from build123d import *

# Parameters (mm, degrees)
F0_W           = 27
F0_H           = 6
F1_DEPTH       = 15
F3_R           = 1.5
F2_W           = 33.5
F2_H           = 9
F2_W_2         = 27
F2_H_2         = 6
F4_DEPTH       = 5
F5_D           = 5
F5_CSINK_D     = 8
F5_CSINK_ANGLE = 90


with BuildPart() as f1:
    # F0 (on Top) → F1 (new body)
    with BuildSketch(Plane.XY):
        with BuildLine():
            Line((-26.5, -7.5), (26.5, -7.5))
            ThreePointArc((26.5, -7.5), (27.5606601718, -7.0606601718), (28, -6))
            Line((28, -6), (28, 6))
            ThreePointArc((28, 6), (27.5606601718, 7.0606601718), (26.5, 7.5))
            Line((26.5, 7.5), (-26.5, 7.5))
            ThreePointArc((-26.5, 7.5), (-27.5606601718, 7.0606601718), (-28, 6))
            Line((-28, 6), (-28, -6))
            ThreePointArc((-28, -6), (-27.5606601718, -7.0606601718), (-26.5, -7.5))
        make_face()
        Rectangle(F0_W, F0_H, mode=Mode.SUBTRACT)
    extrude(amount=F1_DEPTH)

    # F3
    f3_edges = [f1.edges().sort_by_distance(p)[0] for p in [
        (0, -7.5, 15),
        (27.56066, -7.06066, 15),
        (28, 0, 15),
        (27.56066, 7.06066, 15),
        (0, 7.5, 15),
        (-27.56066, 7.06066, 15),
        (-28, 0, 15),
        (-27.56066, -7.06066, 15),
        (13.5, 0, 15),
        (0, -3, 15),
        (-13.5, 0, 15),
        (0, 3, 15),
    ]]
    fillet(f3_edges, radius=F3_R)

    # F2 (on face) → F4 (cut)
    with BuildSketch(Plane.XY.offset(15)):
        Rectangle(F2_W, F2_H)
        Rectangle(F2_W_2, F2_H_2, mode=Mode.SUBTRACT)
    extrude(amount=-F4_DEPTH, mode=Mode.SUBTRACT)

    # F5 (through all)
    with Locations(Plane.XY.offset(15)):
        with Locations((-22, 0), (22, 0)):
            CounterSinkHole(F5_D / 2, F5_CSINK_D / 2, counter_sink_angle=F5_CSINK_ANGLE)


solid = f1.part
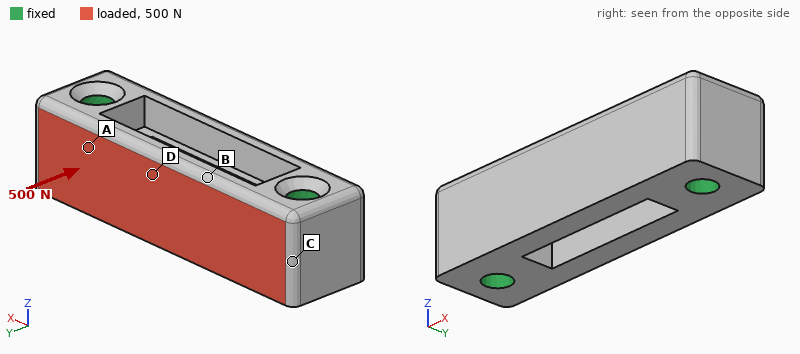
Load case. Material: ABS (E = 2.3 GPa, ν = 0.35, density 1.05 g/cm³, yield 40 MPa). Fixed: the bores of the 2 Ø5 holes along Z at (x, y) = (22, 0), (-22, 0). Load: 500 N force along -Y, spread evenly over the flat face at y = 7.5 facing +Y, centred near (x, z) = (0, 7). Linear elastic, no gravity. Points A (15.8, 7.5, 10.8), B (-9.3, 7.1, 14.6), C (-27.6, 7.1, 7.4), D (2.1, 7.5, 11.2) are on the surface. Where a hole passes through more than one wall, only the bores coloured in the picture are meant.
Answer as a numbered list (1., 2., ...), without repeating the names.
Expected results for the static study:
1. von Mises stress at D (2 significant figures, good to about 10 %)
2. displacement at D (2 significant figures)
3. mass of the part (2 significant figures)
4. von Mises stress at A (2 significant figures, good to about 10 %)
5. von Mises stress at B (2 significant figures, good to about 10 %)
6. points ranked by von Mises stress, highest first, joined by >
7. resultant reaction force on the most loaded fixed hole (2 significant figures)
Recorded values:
1. 9.7 MPa
2. 0.19 mm
3. 9.2 g
4. 7.4 MPa
5. 3.0 MPa
6. D > A > B > C
7. 260 N
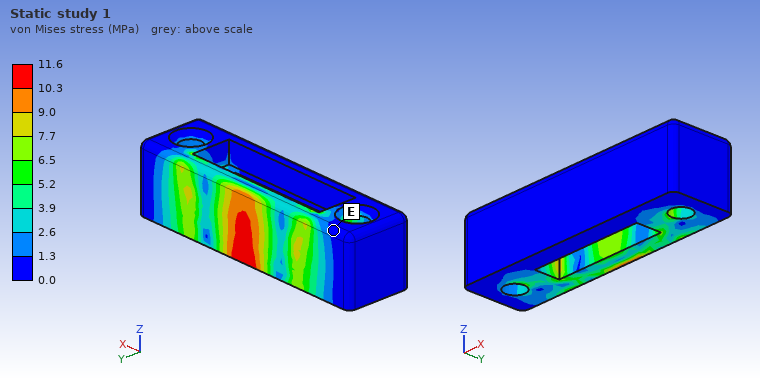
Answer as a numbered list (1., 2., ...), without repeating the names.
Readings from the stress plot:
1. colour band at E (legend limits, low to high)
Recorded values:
1. 0.0 to 1.3 MPa
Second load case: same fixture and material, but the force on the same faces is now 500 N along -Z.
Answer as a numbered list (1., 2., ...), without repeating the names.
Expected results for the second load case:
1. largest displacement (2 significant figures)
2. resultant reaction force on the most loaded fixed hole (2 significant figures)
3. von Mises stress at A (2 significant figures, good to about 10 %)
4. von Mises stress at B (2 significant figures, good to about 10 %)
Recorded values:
1. 0.14 mm
2. 250 N
3. 6.4 MPa
4. 2.9 MPa
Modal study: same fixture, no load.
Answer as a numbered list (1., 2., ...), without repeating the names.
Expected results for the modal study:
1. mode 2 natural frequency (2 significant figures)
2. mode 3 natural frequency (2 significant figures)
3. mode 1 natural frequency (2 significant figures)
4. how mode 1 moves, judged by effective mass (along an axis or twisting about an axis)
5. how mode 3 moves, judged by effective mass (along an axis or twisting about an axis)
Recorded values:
1. 5500 Hz
2. 7900 Hz
3. 5000 Hz
4. along Y
5. twisting about X
